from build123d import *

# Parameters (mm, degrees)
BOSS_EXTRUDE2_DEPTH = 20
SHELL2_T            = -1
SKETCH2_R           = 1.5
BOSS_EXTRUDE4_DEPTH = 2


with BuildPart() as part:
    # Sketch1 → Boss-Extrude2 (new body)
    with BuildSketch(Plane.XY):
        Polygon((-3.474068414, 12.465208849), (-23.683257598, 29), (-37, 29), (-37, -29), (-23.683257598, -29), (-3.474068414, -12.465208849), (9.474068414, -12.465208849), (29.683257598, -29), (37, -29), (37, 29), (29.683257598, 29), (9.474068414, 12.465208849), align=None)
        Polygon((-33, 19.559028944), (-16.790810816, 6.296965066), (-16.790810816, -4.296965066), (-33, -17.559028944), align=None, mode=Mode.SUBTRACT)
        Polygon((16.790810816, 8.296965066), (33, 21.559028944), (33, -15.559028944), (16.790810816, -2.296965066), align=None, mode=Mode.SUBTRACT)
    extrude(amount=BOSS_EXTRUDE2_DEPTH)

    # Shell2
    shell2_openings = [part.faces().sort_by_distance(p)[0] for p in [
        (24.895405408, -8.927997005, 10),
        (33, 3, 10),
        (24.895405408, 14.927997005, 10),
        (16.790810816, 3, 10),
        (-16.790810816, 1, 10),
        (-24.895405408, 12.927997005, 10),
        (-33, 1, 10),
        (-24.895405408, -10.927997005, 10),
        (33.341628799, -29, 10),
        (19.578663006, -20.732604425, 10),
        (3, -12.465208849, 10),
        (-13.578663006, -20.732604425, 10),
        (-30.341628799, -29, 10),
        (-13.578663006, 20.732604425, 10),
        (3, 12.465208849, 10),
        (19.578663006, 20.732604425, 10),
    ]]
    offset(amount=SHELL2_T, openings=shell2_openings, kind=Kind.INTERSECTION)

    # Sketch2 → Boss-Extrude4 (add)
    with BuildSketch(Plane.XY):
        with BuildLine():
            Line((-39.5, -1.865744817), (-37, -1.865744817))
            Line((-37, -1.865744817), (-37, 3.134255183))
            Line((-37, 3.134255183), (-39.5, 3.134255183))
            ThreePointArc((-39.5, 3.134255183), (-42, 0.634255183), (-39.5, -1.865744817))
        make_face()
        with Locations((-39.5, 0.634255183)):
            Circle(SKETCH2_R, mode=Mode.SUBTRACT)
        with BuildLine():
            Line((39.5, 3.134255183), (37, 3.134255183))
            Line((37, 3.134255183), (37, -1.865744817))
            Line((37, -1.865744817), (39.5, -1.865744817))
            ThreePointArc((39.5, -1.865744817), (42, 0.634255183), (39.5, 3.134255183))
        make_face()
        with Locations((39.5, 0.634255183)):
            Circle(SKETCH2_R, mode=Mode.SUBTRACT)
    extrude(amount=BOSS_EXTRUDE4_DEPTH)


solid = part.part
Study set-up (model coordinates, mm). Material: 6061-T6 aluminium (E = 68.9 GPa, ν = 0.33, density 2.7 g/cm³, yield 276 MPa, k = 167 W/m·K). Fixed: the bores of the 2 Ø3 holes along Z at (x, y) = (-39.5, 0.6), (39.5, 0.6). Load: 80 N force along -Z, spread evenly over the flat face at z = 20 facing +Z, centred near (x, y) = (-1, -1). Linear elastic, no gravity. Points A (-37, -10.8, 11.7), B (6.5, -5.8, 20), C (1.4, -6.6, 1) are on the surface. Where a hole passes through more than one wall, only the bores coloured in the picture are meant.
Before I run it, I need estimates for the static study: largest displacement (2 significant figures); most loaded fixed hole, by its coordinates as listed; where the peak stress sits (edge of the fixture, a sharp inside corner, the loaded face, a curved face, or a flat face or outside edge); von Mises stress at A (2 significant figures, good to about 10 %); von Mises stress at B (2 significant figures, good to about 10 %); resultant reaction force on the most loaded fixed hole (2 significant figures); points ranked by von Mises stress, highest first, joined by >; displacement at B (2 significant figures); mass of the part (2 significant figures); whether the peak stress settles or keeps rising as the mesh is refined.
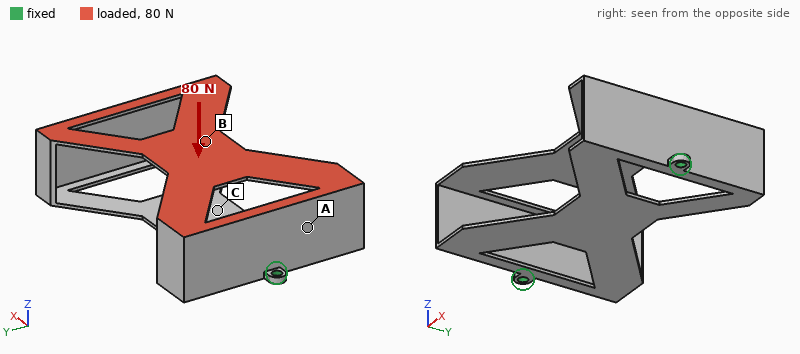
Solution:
0.67 mm
(-39.5, 0.6)
a sharp inside corner
16 MPa
46 MPa
43 N
B > A > C
0.60 mm
20 g
keeps rising
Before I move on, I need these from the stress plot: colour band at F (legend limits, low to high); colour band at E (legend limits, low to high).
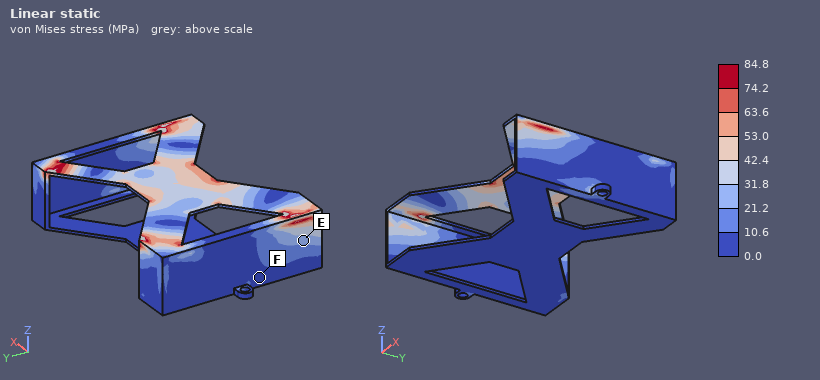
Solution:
0.0 to 10.6 MPa
21.2 to 31.8 MPa
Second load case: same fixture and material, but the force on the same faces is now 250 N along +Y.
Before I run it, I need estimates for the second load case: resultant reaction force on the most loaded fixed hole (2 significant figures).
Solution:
130 N
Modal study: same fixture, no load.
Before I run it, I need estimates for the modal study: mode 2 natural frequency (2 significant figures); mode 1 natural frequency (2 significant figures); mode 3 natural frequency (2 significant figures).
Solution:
790 Hz
790 Hz
860 Hz
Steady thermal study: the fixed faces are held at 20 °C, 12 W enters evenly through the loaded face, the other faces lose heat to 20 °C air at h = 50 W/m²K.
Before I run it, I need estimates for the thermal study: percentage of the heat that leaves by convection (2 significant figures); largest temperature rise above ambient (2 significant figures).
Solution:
64 %
32 K
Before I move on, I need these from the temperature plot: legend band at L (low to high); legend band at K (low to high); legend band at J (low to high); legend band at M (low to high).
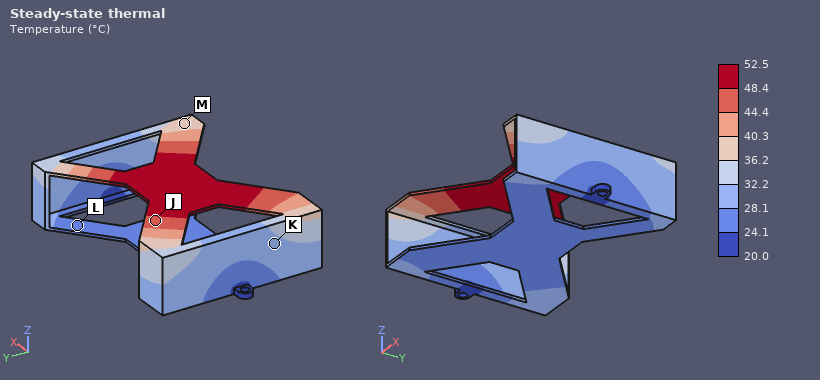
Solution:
24.1 to 28.1 °C
28.1 to 32.2 °C
44.4 to 48.4 °C
36.2 to 40.3 °C
